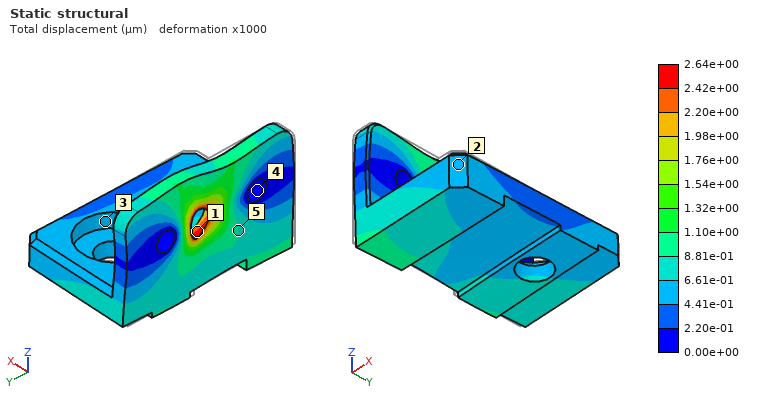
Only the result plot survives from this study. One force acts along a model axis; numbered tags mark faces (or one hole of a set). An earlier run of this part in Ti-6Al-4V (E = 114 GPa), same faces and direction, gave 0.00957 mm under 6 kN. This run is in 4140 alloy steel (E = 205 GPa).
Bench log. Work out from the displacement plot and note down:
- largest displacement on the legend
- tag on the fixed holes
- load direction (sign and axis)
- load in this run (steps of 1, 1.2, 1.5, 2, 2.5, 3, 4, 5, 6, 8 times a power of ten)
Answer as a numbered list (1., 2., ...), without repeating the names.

1. 2.64e+00 µm
2. 4
3. +Y
4. 3 kN
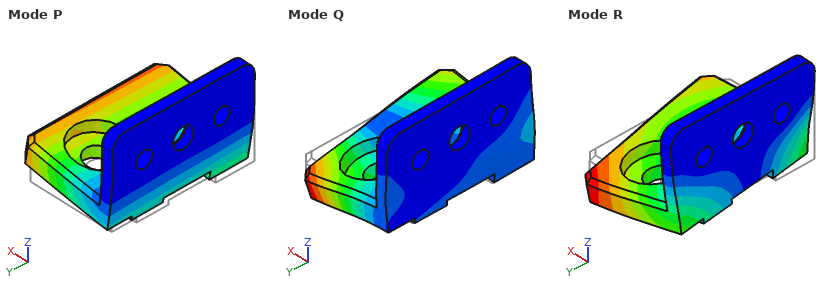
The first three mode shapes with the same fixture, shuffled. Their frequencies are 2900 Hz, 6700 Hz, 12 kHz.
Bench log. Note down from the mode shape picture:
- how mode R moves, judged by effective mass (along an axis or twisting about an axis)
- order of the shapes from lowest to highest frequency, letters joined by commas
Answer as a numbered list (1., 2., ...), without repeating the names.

1. along Y
2. P, R, Q
